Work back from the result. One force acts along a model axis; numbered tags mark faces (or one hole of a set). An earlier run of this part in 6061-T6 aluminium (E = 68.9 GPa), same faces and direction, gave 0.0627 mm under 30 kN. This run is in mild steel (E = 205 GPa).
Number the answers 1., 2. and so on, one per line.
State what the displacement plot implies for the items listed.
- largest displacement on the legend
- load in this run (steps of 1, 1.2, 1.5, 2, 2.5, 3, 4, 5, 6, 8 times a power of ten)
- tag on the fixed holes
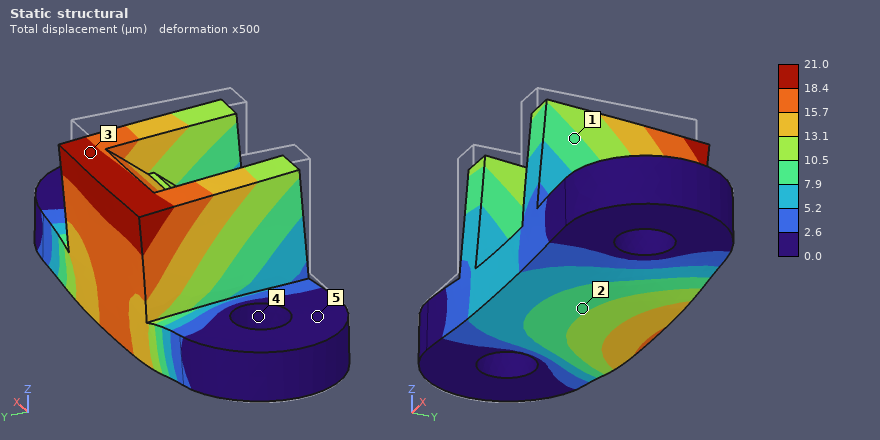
1. 21.0 µm
2. 30 kN
3. 4
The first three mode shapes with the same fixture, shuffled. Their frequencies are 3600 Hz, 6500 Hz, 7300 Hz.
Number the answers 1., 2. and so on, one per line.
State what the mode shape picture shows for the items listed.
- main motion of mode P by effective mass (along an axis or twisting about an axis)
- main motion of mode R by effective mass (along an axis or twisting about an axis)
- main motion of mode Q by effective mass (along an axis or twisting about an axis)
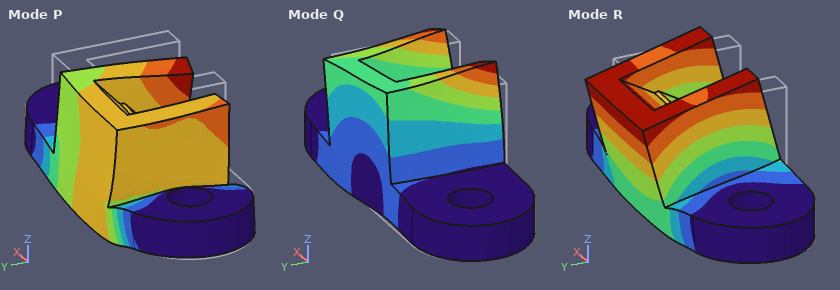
1. along Z
2. along Y
3. along X
